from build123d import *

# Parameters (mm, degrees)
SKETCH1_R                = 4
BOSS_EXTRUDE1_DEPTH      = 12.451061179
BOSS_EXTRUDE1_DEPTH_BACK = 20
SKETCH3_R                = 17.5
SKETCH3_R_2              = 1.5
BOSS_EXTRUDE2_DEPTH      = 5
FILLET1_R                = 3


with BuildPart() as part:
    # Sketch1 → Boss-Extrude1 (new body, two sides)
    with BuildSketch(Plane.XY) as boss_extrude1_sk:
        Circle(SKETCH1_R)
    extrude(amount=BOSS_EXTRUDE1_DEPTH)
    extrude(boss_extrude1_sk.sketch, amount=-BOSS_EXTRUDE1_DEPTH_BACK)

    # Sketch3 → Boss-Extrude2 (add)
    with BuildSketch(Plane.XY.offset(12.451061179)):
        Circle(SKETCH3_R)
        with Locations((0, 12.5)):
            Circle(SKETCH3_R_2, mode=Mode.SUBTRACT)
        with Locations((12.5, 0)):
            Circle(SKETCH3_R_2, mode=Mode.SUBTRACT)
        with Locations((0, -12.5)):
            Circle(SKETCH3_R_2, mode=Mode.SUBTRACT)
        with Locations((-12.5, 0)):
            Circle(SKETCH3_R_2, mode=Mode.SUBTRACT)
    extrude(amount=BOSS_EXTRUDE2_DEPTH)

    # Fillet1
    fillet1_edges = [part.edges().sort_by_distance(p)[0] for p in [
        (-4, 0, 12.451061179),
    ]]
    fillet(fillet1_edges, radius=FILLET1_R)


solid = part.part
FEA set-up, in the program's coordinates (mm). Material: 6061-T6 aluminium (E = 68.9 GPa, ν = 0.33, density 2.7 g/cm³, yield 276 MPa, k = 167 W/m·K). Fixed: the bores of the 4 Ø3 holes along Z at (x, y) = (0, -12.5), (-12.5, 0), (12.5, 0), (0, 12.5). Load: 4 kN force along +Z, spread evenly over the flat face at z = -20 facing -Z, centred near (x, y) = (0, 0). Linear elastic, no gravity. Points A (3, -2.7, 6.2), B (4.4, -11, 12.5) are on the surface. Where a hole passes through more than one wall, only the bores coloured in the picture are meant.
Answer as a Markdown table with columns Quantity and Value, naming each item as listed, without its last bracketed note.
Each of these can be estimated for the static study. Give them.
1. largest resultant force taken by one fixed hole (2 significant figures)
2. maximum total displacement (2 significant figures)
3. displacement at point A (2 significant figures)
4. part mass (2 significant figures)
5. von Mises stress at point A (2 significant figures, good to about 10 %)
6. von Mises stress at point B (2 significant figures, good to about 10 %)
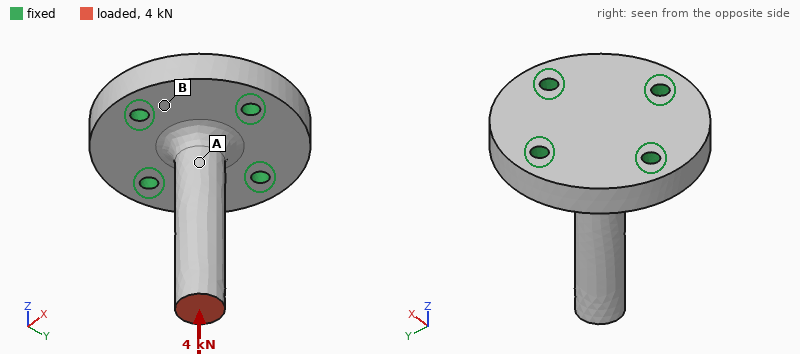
| Quantity | Value |
|---|---|
| largest resultant force taken by one fixed hole | 1.0 kN |
| maximum total displacement | 51 µm |
| displacement at point A | 21 µm |
| part mass | 17 g |
| von Mises stress at point A | 77 MPa |
| von Mises stress at point B | 20 MPa |
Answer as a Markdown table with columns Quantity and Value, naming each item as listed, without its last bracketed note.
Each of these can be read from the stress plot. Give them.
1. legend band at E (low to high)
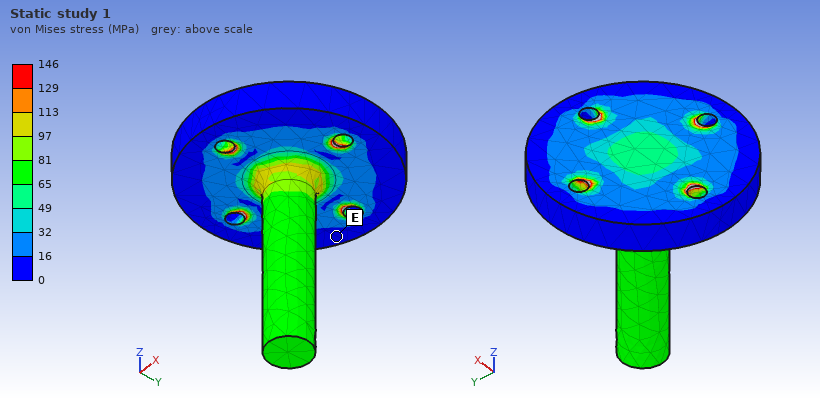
| Quantity | Value |
|---|---|
| legend band at E | 0 to 16 MPa |
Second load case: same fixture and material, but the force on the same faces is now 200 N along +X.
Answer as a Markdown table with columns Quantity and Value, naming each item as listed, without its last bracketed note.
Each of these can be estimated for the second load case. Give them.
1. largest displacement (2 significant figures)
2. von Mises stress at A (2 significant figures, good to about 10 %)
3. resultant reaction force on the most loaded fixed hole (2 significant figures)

| Quantity | Value |
|---|---|
| largest displacement | 0.18 mm |
| von Mises stress at A | 77 MPa |
| resultant reaction force on the most loaded fixed hole | 320 N |
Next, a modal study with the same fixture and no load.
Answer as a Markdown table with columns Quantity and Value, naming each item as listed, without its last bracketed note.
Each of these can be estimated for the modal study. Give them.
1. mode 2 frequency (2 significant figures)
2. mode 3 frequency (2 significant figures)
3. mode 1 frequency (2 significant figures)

| Quantity | Value |
|---|---|
| mode 2 frequency | 5000 Hz |
| mode 3 frequency | 24 kHz |
| mode 1 frequency | 5000 Hz |
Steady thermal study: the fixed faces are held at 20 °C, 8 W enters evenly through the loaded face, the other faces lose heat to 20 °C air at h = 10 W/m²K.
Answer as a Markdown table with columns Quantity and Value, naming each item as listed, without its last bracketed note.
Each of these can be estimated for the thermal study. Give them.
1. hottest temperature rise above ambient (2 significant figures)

| Quantity | Value |
|---|---|
| hottest temperature rise above ambient | 33 K |
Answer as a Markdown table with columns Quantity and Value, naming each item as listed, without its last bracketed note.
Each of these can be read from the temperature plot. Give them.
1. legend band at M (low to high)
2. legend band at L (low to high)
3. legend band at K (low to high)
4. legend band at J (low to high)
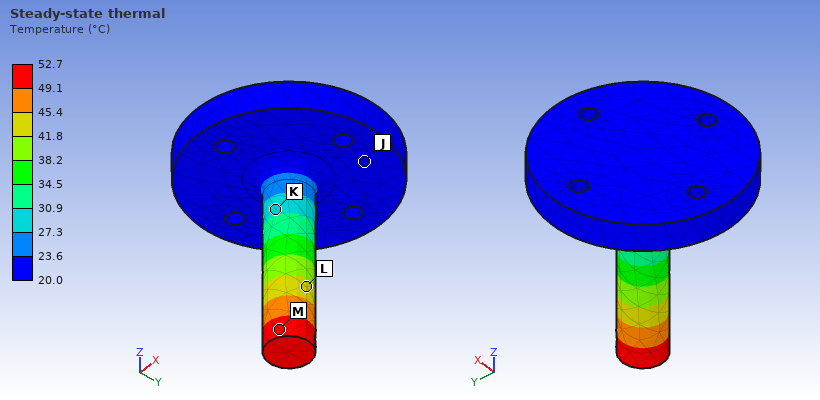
| Quantity | Value |
|---|---|
| legend band at M | 49.1 to 52.7 °C |
| legend band at L | 41.8 to 45.4 °C |
| legend band at K | 27.3 to 30.9 °C |
| legend band at J | 20.0 to 23.6 °C |
